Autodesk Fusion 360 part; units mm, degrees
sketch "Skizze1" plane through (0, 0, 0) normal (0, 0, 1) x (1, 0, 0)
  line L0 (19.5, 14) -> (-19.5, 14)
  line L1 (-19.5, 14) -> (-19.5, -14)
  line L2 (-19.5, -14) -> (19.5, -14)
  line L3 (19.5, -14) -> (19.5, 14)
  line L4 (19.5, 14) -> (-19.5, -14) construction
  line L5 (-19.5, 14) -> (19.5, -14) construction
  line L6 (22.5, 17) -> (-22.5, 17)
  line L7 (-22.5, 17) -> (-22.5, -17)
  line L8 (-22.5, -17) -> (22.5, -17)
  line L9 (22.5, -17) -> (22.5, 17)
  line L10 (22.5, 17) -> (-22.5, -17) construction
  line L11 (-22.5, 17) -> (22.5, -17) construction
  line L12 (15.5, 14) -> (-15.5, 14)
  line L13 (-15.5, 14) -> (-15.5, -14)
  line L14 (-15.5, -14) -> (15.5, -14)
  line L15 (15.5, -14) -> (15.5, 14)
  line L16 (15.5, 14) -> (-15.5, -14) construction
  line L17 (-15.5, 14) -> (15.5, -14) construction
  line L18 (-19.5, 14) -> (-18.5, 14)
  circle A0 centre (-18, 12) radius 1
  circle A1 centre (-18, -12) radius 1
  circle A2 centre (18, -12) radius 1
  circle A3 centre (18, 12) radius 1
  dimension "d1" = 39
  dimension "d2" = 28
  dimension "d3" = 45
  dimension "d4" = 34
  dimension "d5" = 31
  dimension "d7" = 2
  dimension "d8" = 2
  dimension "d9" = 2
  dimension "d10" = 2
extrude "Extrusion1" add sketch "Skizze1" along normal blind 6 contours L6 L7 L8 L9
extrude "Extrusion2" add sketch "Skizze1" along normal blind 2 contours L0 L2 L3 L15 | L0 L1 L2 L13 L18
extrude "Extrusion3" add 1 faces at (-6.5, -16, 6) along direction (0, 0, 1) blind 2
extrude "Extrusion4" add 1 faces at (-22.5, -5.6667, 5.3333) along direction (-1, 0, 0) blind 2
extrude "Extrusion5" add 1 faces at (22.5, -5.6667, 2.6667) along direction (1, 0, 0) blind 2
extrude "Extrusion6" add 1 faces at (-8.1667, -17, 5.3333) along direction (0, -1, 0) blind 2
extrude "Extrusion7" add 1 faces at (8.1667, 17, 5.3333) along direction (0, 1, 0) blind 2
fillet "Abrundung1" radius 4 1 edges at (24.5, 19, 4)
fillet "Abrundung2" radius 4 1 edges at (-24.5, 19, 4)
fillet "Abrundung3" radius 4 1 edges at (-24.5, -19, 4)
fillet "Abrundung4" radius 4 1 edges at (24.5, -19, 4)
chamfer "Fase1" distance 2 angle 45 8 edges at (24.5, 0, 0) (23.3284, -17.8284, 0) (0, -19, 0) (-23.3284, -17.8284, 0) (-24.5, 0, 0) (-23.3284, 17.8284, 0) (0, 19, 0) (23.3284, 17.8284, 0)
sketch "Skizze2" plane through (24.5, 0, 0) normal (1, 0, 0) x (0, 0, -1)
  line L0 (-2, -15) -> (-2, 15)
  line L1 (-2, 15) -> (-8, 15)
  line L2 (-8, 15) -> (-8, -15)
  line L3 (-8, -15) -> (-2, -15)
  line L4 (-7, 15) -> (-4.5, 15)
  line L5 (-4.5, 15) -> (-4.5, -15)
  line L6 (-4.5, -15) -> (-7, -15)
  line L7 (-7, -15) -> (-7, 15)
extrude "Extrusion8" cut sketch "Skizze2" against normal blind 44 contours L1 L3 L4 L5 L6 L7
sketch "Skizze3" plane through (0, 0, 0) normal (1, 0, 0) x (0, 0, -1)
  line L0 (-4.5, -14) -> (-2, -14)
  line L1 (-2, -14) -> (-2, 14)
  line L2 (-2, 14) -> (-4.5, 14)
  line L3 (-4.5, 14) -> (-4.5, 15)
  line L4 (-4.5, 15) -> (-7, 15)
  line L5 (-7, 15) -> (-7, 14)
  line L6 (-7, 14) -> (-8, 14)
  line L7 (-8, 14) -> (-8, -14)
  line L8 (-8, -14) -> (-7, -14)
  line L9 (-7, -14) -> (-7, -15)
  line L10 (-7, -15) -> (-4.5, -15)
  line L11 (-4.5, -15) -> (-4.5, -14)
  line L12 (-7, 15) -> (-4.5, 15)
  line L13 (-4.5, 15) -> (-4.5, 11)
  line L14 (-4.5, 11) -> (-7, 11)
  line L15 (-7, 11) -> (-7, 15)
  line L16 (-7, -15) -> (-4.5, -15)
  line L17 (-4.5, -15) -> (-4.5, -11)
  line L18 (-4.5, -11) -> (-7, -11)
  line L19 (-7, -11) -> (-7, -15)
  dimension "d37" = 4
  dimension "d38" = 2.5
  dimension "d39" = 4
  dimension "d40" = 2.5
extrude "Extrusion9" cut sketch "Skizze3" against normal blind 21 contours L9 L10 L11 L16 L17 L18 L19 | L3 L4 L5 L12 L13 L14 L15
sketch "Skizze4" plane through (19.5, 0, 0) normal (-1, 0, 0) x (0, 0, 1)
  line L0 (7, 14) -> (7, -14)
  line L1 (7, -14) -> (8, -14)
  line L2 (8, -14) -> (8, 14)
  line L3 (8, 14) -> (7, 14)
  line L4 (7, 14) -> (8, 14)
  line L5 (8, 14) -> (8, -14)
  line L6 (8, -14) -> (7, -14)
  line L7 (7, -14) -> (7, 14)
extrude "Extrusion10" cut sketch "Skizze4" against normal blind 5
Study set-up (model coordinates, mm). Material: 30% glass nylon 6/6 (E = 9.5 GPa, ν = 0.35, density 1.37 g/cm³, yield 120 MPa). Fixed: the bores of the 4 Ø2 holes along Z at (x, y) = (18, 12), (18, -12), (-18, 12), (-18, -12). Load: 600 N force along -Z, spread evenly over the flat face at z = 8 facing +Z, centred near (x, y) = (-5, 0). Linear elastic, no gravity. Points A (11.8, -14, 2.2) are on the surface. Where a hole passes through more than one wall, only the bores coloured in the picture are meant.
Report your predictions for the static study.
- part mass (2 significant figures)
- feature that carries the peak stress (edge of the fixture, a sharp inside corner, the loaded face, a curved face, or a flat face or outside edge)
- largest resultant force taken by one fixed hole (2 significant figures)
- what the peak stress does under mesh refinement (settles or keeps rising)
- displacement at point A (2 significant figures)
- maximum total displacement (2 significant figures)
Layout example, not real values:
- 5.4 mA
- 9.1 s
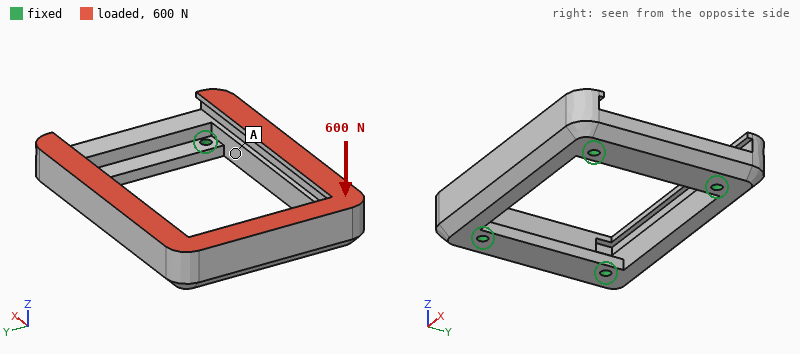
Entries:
- 7.4 g
- edge of the fixture
- 190 N
- keeps rising
- 40 µm
- 97 µm
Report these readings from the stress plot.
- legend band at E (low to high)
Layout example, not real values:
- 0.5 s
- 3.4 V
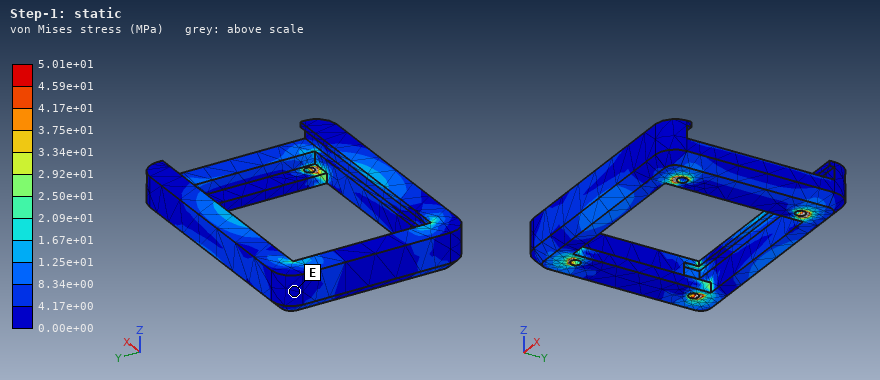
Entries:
- 0.00e+00 to 4.17e+00 MPa
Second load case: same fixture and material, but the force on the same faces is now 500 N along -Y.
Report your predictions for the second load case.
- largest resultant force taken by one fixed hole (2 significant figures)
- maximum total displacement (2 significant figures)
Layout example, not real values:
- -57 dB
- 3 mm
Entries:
- 200 N
- 0.17 mm
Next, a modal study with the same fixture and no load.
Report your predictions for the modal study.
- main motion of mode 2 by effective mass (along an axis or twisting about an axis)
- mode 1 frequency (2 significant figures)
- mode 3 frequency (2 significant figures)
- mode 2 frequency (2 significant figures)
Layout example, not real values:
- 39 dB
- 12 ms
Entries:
- along Y
- 4800 Hz
- 8500 Hz
- 5400 Hz
